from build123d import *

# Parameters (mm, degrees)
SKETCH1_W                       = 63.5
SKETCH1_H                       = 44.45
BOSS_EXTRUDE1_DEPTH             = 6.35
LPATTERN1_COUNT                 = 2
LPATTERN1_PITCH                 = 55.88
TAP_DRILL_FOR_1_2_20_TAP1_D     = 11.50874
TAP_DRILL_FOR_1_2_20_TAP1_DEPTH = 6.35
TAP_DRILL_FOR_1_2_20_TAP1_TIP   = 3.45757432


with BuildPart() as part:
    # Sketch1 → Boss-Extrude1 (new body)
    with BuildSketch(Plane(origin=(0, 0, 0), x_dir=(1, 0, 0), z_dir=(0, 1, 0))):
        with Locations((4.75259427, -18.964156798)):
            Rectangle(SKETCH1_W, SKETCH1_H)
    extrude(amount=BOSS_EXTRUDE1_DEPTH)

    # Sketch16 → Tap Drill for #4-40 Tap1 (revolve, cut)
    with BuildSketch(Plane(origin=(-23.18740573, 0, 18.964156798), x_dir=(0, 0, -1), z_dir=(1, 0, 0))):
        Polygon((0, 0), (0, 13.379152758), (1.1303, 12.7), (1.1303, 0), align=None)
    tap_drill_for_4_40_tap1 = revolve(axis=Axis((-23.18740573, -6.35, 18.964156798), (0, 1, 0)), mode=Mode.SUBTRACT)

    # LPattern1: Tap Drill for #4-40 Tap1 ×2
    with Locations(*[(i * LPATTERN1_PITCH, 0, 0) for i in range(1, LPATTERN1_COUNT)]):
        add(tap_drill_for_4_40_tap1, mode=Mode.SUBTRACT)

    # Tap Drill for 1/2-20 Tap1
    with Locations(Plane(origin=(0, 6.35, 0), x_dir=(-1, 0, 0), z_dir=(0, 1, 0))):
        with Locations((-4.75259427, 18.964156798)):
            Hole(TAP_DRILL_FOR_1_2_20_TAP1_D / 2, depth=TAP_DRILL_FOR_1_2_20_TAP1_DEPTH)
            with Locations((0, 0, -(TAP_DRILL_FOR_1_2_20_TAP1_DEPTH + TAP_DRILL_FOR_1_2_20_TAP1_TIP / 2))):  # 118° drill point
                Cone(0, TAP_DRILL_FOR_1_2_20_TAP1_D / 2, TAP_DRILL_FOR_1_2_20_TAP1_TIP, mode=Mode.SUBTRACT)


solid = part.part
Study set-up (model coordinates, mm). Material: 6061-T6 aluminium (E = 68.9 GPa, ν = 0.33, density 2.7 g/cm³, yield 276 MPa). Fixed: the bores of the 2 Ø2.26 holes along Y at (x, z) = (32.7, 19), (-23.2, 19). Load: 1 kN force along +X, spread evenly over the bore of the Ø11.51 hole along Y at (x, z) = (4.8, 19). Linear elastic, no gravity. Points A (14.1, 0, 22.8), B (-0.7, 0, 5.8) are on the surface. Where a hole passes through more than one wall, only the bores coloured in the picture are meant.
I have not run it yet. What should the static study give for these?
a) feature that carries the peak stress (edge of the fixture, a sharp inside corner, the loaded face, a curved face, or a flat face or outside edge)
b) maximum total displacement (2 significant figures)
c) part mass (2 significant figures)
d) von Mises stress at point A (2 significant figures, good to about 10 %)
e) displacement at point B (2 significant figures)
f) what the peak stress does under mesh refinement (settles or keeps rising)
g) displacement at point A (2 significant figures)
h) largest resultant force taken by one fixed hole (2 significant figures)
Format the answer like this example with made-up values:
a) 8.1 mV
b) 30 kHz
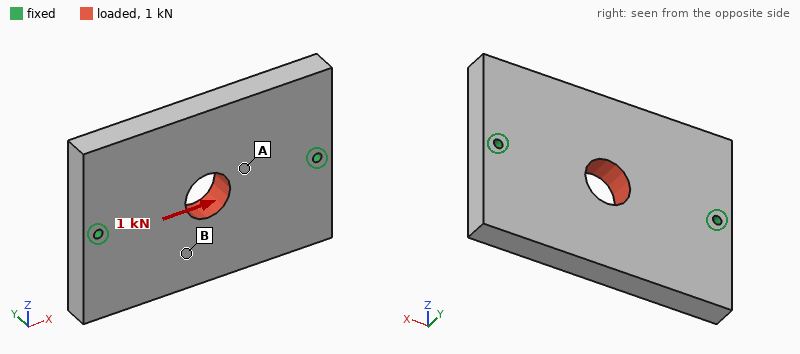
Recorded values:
a) edge of the fixture
b) 2.1 µm
c) 46 g
d) 4.6 MPa
e) 1.5 µm
f) keeps rising
g) 1.7 µm
h) 500 N
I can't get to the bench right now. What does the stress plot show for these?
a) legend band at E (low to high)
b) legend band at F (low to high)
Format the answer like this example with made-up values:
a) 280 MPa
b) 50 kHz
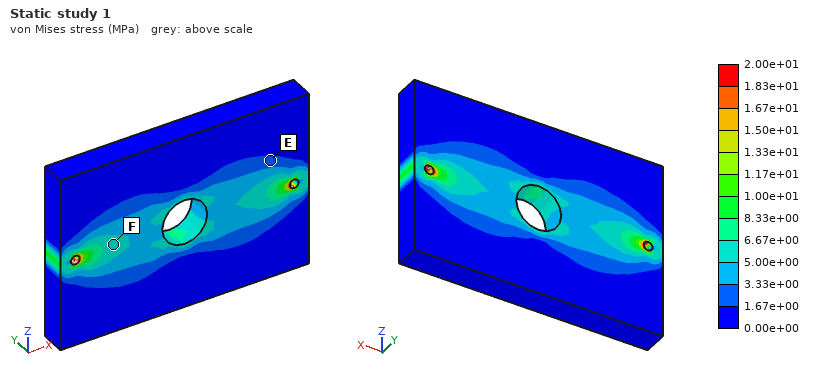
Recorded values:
a) 1.67e+00 to 3.33e+00 MPa
b) 5.00e+00 to 6.67e+00 MPa
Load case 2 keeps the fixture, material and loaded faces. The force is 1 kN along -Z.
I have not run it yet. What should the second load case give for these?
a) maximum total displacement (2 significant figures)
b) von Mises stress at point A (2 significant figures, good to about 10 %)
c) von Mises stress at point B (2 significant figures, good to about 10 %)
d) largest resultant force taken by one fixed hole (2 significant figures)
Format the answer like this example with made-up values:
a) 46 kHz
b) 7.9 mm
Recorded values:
a) 3.8 µm
b) 4.1 MPa
c) 4.1 MPa
d) 500 N
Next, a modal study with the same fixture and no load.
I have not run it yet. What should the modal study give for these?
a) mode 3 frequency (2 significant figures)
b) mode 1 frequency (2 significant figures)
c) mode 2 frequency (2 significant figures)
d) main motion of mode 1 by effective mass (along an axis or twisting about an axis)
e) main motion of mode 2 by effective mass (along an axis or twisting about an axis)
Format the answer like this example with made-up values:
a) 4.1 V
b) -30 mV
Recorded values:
a) 9800 Hz
b) 4500 Hz
c) 5800 Hz
d) twisting about X
e) along Y
